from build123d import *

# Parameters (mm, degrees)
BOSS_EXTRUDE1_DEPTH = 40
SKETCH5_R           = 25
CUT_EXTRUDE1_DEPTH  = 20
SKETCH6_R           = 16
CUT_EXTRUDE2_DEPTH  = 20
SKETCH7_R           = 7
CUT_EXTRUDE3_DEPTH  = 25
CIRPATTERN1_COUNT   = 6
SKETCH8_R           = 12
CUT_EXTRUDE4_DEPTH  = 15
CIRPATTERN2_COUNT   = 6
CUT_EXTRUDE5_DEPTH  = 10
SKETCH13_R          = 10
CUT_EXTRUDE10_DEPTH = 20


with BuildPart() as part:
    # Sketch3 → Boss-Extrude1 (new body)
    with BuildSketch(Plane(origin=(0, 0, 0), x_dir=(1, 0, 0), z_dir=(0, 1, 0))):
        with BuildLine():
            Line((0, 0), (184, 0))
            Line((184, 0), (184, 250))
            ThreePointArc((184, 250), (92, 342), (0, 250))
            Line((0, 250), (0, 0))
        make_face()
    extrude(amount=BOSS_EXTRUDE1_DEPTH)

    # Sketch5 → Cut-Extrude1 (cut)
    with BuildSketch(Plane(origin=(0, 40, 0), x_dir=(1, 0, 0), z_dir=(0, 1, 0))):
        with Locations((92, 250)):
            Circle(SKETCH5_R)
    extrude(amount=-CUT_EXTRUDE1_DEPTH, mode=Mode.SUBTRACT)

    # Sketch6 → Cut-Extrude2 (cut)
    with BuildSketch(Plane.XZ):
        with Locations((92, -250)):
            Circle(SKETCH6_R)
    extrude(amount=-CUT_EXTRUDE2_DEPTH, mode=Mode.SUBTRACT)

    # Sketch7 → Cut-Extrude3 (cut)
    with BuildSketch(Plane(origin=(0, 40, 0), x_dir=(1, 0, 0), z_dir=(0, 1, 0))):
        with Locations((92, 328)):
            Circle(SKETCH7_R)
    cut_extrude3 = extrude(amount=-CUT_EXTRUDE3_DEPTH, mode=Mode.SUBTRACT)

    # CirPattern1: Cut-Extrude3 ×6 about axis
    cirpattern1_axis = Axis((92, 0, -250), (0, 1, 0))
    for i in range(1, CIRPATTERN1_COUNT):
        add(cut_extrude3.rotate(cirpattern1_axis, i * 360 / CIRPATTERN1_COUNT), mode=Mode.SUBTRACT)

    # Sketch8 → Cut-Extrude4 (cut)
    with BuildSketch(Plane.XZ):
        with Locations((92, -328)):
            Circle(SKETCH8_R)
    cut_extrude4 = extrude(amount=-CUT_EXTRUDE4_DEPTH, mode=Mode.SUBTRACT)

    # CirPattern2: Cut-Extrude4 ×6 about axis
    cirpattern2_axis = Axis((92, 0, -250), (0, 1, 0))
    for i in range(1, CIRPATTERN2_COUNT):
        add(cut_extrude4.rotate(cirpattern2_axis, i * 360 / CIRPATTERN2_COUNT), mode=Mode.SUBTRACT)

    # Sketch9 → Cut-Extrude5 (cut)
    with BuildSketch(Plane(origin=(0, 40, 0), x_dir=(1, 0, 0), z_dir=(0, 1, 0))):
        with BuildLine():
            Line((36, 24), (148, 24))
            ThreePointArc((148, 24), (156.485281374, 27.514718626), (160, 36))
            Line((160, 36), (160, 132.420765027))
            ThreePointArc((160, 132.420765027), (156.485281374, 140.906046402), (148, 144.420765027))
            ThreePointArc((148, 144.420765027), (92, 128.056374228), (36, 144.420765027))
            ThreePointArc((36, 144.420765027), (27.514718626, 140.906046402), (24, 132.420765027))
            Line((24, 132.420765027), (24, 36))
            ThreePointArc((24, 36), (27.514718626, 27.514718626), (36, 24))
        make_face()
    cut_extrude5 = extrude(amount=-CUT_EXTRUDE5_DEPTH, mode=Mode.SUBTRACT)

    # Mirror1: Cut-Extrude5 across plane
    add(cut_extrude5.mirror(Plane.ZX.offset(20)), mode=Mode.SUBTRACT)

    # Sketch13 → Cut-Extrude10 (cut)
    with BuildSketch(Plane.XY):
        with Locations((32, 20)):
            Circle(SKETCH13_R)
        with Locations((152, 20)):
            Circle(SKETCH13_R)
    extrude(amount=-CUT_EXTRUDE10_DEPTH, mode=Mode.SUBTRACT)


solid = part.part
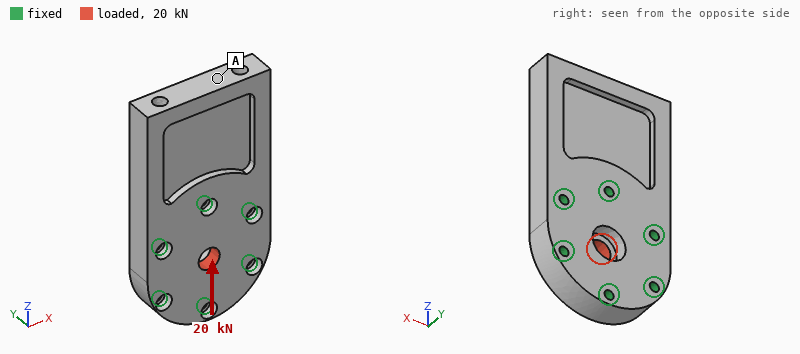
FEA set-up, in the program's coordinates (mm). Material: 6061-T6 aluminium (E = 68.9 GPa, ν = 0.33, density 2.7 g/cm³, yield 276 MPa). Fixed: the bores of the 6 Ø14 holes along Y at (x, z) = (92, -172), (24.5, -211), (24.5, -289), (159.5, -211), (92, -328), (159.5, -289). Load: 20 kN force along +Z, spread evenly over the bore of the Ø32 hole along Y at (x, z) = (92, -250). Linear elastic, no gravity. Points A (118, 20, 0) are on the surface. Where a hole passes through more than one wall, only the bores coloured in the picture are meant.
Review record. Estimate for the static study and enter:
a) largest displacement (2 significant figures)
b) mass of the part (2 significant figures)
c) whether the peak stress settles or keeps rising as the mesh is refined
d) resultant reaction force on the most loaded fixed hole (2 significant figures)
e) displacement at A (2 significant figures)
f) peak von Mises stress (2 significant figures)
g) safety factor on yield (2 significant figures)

7.0 µm
5.2 kg
settles
5.0 kN
4.7 µm
19 MPa
15
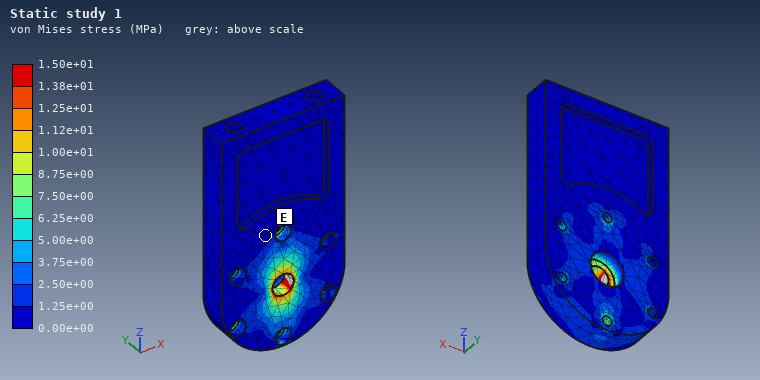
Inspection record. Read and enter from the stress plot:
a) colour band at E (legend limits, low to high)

0.00e+00 to 1.25e+00 MPa
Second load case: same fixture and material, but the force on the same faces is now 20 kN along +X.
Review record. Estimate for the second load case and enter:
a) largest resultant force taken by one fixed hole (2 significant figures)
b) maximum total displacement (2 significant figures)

4.5 kN
7.0 µm
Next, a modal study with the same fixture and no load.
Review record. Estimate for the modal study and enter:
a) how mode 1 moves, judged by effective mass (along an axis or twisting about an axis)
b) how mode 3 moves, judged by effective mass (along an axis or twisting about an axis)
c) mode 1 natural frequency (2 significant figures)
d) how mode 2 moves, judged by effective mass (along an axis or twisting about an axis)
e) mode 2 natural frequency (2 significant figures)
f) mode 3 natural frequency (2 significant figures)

along Y
along X
750 Hz
twisting about Z
1300 Hz
2400 Hz
